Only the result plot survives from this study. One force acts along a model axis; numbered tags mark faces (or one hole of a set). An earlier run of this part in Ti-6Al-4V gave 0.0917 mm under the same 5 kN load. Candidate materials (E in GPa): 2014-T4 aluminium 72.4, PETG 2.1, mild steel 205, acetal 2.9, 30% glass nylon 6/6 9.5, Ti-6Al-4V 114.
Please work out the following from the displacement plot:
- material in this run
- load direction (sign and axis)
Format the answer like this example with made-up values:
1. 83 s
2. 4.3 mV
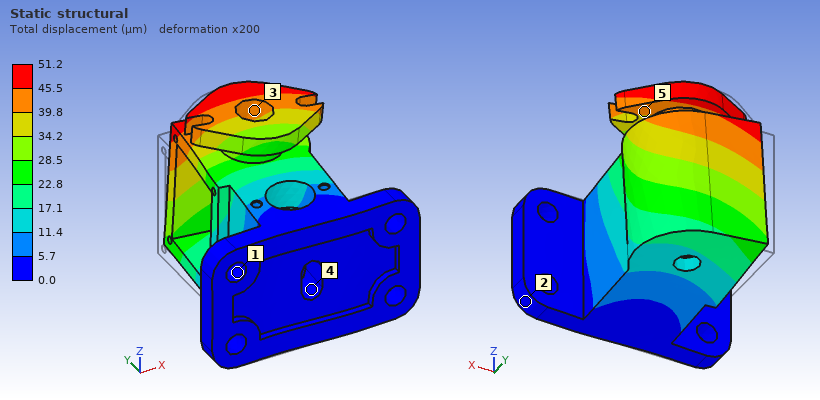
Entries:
1. mild steel
2. +X
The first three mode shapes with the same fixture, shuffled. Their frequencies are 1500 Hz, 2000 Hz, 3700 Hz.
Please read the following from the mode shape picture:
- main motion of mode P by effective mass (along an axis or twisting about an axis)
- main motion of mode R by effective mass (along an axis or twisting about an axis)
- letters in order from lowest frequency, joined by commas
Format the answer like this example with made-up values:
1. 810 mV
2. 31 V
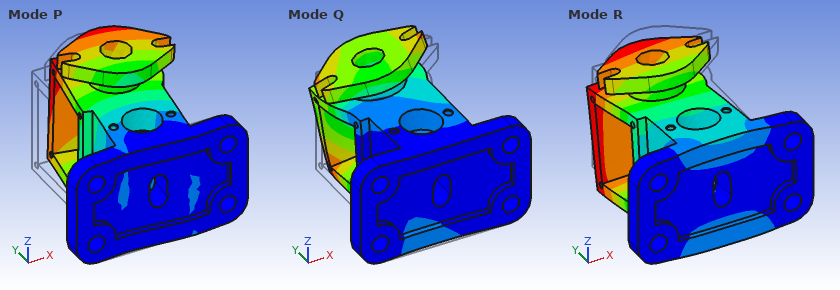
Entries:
1. along X
2. along Z
3. R, P, Q
